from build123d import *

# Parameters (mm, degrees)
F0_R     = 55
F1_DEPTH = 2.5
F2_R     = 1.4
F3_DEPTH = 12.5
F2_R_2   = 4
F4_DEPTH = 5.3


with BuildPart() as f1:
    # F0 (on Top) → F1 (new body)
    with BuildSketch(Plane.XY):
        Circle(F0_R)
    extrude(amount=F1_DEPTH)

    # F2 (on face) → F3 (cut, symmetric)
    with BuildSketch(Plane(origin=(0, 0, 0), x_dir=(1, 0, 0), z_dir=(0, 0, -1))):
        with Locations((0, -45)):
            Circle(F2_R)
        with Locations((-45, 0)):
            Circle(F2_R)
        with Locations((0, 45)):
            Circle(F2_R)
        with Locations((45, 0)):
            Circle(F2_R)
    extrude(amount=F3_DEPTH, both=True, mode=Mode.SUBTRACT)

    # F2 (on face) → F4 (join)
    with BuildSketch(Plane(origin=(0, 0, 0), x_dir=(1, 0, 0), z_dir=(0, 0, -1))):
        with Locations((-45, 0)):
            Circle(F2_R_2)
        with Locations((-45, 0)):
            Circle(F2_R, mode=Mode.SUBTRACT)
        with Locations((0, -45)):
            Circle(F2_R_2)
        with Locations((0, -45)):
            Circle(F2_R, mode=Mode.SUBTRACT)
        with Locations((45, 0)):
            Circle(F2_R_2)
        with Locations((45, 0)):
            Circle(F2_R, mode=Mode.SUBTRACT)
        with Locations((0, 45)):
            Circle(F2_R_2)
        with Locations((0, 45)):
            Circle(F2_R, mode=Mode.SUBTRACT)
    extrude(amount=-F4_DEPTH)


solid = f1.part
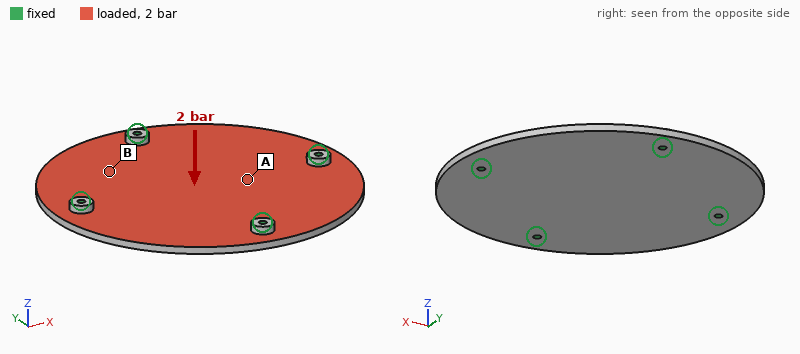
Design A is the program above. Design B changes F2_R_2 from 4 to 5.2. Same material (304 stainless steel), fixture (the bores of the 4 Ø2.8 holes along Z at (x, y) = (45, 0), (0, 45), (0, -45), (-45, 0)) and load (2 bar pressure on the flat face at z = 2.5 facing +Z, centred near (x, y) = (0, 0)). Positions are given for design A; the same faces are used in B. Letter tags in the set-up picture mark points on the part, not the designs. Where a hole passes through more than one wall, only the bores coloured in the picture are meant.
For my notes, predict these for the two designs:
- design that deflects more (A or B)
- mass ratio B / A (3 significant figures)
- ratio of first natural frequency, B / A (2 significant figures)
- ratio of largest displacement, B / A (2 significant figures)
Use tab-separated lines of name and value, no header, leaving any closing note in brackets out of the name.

design that deflects more	A
mass ratio B / A	1.02
ratio of first natural frequency, B / A	1.1
ratio of largest displacement, B / A	0.89
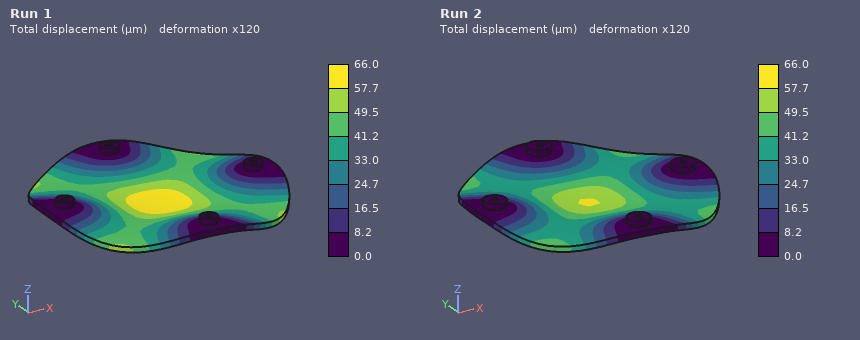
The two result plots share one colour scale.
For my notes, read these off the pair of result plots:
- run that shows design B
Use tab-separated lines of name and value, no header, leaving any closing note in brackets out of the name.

run that shows design B	Run 2
